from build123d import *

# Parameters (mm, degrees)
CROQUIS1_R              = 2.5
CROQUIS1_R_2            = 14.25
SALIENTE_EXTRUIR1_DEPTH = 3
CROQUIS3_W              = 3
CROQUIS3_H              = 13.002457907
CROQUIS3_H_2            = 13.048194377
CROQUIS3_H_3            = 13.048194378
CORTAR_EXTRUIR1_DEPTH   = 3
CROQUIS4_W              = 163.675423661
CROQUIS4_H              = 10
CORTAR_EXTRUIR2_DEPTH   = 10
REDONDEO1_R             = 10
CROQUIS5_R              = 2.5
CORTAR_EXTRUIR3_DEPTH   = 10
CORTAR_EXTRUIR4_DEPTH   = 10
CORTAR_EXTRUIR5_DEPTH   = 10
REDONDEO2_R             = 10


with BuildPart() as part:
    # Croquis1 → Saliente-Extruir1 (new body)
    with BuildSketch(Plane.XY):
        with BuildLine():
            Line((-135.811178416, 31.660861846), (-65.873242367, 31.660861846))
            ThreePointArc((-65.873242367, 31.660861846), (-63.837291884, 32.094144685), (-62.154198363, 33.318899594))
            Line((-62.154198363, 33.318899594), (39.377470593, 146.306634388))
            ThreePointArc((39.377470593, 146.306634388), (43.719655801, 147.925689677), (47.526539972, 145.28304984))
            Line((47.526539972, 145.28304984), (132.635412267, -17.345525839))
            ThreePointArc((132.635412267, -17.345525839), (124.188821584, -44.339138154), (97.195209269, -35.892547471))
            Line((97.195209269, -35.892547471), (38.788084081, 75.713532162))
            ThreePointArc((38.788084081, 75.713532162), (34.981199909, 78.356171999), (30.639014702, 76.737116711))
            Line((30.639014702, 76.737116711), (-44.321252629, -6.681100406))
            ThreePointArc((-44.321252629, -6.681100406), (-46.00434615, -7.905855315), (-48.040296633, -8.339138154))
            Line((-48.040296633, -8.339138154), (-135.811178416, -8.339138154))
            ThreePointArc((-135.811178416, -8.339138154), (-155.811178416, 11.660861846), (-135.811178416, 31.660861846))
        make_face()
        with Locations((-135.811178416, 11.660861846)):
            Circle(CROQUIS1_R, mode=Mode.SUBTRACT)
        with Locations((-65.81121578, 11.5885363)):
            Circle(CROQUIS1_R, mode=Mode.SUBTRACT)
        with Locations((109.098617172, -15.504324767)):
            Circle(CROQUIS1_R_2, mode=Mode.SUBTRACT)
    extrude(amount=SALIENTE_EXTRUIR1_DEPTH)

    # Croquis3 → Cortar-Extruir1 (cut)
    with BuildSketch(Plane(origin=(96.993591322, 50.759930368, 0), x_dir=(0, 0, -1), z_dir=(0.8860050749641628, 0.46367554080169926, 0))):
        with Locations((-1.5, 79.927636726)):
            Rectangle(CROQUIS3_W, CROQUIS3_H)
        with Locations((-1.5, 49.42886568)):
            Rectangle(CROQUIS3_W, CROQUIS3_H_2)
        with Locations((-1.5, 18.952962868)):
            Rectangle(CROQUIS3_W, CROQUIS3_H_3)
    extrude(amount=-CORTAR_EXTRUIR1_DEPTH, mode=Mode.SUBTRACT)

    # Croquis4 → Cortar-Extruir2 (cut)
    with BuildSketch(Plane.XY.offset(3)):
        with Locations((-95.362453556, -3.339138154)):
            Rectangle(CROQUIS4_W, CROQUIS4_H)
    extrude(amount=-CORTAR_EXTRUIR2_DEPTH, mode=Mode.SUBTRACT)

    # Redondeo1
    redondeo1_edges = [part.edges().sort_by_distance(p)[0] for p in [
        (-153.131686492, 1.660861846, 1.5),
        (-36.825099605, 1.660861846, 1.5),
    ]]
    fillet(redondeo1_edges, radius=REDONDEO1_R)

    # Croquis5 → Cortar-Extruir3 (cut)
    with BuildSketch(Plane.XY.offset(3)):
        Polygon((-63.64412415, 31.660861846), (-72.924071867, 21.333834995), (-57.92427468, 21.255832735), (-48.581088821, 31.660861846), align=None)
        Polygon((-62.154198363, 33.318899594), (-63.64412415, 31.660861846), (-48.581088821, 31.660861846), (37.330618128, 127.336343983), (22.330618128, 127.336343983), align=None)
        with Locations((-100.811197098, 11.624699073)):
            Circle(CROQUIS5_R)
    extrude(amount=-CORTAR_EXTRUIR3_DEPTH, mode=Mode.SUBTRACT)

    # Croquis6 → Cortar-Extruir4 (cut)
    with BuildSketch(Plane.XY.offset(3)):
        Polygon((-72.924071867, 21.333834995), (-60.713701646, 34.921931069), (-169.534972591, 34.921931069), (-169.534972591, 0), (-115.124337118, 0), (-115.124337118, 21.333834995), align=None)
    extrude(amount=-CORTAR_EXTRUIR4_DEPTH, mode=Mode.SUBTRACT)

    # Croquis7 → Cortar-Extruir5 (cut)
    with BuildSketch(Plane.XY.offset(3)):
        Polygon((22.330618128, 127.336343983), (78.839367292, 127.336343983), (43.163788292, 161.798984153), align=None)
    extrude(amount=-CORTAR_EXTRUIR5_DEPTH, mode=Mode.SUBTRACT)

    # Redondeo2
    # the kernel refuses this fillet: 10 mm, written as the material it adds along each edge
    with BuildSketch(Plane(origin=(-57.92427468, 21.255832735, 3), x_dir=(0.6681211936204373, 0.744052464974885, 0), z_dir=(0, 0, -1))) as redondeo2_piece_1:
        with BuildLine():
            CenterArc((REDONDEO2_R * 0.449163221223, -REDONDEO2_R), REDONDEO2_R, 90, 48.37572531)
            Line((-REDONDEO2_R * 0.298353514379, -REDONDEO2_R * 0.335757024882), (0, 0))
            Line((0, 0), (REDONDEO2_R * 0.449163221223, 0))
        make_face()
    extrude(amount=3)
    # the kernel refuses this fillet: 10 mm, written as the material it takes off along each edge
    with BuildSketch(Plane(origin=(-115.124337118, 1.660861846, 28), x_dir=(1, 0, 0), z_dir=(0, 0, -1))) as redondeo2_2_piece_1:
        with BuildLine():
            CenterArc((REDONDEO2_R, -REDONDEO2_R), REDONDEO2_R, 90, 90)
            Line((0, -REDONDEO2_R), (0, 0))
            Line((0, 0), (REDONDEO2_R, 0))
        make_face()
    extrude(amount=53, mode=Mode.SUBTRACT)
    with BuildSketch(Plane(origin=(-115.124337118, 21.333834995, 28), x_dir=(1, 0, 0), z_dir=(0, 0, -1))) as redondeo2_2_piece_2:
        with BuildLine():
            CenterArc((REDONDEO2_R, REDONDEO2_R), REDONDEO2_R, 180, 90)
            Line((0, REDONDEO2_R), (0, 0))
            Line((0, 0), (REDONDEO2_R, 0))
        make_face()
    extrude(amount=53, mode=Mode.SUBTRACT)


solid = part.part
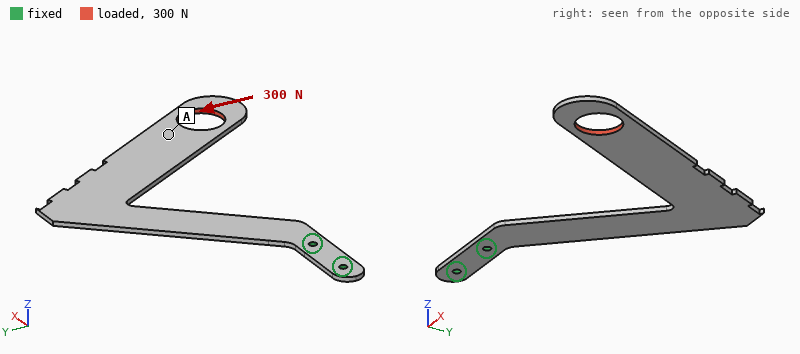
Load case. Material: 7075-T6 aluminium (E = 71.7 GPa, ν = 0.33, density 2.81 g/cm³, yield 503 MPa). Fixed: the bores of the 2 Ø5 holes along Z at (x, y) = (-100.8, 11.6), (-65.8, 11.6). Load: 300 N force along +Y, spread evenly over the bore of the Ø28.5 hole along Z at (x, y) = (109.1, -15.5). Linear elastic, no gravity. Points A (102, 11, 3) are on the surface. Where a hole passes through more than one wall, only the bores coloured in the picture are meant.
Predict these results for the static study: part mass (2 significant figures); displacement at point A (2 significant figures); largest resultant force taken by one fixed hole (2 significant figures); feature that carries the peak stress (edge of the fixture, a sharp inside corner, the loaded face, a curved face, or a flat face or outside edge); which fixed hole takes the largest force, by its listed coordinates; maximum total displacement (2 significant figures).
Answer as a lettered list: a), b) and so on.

a) 94 g
b) 2.6 mm
c) 1.2 kN
d) edge of the fixture
e) (-65.8, 11.6)
f) 3.5 mm
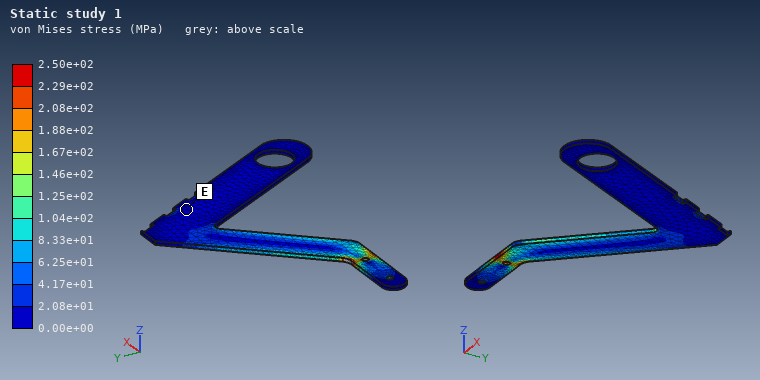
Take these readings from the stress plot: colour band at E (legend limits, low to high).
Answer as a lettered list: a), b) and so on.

a) 0.00e+00 to 2.08e+01 MPa
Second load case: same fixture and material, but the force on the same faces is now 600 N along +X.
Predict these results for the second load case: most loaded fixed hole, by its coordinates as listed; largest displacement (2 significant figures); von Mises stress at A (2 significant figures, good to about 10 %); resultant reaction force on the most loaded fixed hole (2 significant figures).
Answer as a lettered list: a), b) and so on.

a) (-65.8, 11.6)
b) 3.0 mm
c) 14 MPa
d) 610 N
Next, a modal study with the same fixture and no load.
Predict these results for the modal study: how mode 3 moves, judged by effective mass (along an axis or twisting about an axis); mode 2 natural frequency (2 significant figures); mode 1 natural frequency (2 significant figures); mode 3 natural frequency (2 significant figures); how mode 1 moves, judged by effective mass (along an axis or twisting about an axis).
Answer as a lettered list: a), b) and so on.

a) along Y
b) 81 Hz
c) 38 Hz
d) 250 Hz
e) along Z
